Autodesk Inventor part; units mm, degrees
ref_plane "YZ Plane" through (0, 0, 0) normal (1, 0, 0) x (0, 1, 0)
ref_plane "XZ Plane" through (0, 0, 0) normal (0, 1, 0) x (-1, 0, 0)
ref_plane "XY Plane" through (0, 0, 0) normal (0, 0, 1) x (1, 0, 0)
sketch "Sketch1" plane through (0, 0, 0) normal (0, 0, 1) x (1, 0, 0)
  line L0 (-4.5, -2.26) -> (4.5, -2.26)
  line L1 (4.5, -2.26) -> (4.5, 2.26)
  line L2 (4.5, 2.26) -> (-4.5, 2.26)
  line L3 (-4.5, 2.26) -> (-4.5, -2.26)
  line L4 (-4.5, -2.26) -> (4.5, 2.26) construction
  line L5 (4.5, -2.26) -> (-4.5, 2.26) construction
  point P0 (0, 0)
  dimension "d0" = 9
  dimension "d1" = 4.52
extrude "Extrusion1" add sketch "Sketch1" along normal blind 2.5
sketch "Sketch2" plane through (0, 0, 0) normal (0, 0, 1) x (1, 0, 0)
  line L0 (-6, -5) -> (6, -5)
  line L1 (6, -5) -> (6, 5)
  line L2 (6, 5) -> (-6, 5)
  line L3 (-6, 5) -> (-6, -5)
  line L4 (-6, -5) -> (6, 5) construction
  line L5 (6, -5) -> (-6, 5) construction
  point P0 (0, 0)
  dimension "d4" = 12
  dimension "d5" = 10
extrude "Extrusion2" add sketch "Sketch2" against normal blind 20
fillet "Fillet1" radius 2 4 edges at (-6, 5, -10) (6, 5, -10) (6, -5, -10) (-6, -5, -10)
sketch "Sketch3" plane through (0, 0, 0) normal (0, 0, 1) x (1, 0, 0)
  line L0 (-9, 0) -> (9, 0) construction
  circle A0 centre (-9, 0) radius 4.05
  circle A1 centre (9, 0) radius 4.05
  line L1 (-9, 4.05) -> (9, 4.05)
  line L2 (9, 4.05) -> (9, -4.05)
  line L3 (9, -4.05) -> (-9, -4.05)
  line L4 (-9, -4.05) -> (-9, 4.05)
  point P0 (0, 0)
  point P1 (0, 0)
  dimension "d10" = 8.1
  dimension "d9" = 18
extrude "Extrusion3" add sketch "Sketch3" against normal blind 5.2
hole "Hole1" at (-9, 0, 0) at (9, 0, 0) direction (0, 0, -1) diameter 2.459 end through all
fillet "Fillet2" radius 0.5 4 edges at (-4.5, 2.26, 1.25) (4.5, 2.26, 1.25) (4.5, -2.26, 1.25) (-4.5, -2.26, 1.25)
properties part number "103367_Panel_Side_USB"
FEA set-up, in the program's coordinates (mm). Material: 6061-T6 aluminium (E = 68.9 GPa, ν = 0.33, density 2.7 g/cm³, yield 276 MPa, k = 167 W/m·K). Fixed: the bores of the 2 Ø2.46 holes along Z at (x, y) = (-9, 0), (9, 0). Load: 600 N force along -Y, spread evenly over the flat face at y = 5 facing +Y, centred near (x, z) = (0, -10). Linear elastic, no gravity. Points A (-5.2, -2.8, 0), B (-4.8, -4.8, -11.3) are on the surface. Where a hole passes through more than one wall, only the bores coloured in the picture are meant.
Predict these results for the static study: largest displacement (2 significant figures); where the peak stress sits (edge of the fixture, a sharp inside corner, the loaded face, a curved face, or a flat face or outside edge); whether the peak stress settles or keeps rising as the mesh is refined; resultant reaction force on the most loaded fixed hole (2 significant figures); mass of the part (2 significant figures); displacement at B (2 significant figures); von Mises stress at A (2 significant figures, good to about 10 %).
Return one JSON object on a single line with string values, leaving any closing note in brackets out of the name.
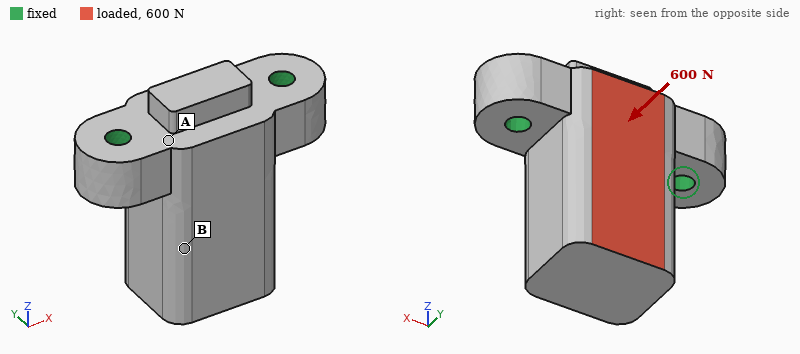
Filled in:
{"largest displacement": "35 µm", "where the peak stress sits": "edge of the fixture", "whether the peak stress settles or keeps rising as the mesh is refined": "keeps rising", "resultant reaction force on the most loaded fixed hole": "300 N", "mass of the part": "7.8 g", "displacement at B": "19 µm", "von Mises stress at A": "28 MPa"}
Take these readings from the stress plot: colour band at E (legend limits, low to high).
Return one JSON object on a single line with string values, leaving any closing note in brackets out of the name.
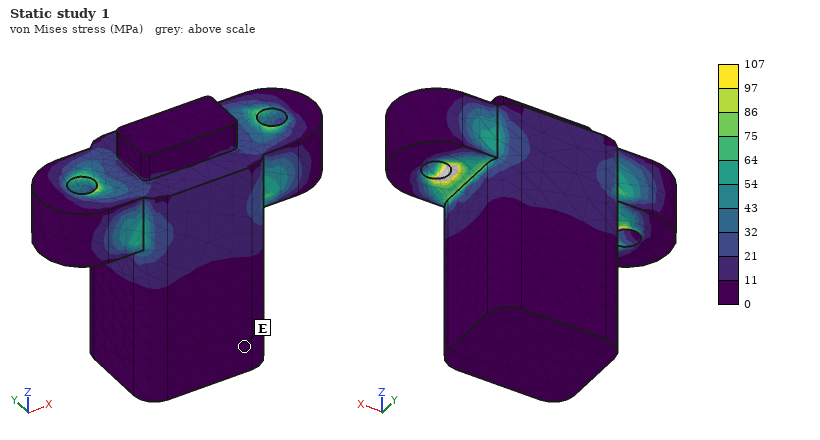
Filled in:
{"colour band at E": "0 to 11 MPa"}
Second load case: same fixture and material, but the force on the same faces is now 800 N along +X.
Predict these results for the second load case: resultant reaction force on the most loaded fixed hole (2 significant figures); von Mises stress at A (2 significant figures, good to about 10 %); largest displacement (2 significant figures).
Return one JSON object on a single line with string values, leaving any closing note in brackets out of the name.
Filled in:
{"resultant reaction force on the most loaded fixed hole": "600 N", "von Mises stress at A": "13 MPa", "largest displacement": "13 µm"}
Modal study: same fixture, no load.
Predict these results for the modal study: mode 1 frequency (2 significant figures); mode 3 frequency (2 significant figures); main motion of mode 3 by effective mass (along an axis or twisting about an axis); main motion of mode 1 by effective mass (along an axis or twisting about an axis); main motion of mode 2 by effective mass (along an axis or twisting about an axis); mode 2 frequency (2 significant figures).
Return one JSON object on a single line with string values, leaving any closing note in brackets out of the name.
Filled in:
{"mode 1 frequency": "10 kHz", "mode 3 frequency": "34 kHz", "main motion of mode 3 by effective mass": "along Z", "main motion of mode 1 by effective mass": "along Y", "main motion of mode 2 by effective mass": "along X", "mode 2 frequency": "21 kHz"}
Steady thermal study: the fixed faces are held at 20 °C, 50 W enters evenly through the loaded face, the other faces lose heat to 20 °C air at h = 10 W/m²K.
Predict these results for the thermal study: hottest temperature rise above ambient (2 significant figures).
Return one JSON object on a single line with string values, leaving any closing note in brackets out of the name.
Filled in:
{"hottest temperature rise above ambient": "38 K"}
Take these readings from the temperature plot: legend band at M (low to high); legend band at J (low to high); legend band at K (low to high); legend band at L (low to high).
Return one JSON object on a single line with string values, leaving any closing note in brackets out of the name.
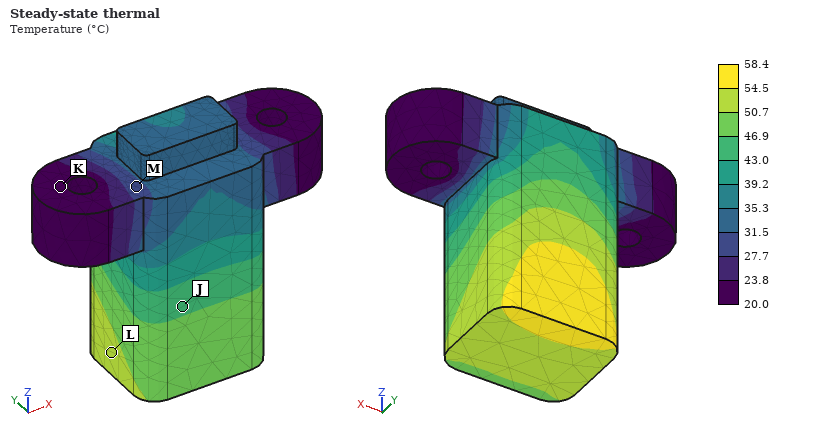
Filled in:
{"legend band at M": "27.7 to 31.5 °C", "legend band at J": "43.0 to 46.9 °C", "legend band at K": "20.0 to 23.8 °C", "legend band at L": "50.7 to 54.5 °C"}
